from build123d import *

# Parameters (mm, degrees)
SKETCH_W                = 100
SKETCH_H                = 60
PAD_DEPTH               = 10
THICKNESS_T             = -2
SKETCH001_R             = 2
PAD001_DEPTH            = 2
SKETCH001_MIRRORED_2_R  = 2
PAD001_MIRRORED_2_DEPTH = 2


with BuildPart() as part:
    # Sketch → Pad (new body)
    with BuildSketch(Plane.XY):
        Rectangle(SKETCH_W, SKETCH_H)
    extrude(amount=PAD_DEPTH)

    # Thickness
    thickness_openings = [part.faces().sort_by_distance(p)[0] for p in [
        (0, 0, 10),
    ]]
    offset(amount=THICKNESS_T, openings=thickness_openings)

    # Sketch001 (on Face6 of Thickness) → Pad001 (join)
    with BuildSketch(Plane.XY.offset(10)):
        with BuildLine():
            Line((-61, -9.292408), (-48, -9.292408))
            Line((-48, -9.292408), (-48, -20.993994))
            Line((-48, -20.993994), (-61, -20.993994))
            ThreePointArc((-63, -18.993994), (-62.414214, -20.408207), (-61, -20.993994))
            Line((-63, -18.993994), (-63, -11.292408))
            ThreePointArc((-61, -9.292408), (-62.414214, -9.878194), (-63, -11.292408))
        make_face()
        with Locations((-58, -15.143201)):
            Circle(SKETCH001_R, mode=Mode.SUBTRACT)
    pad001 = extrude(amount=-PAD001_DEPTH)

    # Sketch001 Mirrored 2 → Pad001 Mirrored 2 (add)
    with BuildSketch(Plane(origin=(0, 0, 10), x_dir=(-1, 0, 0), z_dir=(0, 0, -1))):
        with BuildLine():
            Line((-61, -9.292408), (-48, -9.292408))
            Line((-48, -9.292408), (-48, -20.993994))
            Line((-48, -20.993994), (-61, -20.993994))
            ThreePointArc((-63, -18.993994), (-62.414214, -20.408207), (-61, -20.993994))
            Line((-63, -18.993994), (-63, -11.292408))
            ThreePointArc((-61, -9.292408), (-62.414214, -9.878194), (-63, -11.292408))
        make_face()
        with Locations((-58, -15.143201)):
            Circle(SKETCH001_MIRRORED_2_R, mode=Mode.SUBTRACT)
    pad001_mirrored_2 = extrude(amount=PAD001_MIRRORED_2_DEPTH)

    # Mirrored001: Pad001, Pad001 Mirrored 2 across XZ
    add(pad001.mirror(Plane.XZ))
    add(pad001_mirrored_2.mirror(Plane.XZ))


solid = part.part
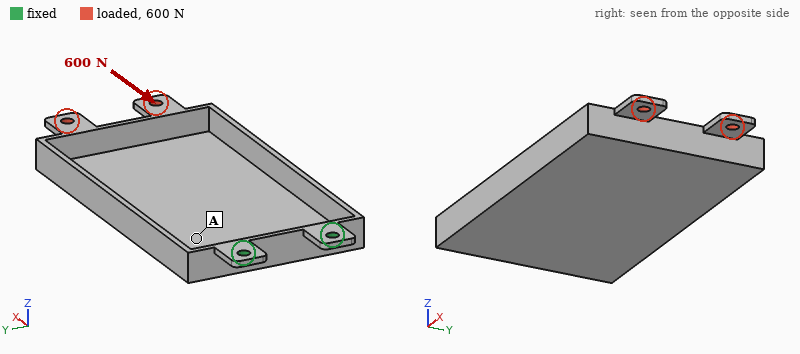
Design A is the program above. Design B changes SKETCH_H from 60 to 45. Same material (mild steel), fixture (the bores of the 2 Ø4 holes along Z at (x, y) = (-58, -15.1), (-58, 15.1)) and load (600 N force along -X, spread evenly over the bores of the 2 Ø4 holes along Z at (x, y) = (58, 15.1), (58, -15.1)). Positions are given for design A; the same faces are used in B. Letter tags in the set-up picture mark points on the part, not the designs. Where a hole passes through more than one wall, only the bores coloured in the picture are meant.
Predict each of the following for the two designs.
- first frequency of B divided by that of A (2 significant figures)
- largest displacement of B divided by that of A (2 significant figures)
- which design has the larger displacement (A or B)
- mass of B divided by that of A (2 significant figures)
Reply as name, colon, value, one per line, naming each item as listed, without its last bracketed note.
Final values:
first frequency of B divided by that of A: 1.2
largest displacement of B divided by that of A: 0.42
which design has the larger displacement: A
mass of B divided by that of A: 0.81
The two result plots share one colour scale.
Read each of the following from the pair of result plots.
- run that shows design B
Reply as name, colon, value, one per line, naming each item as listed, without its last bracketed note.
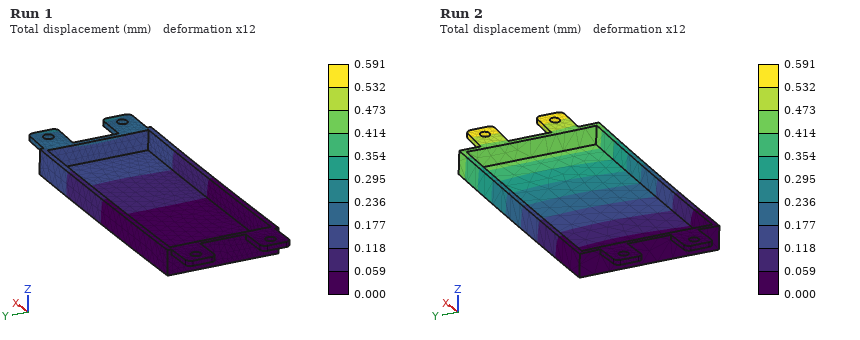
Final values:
run that shows design B: Run 1
